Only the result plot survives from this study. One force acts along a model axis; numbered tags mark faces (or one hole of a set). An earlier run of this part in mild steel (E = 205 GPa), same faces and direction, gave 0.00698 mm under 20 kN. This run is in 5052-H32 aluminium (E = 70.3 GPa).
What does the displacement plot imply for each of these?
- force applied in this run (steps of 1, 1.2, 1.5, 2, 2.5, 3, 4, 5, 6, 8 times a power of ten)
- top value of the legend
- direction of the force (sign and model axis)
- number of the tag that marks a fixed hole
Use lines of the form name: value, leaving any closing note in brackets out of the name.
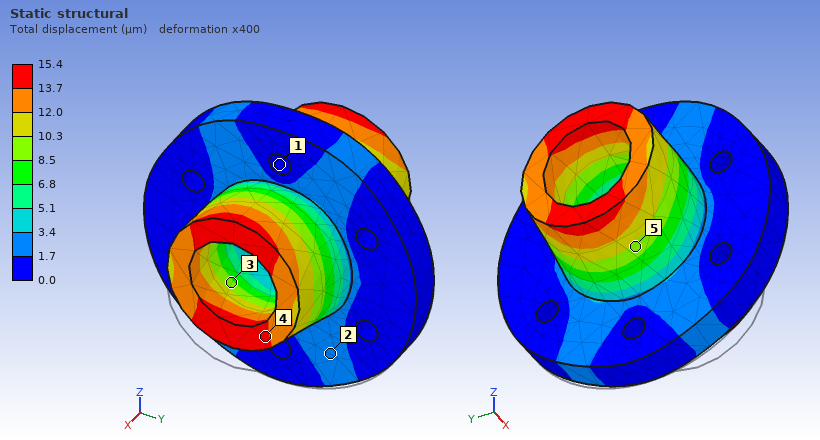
force applied in this run: 15 kN
top value of the legend: 15.4 µm
direction of the force: +Z
number of the tag that marks a fixed hole: 1
